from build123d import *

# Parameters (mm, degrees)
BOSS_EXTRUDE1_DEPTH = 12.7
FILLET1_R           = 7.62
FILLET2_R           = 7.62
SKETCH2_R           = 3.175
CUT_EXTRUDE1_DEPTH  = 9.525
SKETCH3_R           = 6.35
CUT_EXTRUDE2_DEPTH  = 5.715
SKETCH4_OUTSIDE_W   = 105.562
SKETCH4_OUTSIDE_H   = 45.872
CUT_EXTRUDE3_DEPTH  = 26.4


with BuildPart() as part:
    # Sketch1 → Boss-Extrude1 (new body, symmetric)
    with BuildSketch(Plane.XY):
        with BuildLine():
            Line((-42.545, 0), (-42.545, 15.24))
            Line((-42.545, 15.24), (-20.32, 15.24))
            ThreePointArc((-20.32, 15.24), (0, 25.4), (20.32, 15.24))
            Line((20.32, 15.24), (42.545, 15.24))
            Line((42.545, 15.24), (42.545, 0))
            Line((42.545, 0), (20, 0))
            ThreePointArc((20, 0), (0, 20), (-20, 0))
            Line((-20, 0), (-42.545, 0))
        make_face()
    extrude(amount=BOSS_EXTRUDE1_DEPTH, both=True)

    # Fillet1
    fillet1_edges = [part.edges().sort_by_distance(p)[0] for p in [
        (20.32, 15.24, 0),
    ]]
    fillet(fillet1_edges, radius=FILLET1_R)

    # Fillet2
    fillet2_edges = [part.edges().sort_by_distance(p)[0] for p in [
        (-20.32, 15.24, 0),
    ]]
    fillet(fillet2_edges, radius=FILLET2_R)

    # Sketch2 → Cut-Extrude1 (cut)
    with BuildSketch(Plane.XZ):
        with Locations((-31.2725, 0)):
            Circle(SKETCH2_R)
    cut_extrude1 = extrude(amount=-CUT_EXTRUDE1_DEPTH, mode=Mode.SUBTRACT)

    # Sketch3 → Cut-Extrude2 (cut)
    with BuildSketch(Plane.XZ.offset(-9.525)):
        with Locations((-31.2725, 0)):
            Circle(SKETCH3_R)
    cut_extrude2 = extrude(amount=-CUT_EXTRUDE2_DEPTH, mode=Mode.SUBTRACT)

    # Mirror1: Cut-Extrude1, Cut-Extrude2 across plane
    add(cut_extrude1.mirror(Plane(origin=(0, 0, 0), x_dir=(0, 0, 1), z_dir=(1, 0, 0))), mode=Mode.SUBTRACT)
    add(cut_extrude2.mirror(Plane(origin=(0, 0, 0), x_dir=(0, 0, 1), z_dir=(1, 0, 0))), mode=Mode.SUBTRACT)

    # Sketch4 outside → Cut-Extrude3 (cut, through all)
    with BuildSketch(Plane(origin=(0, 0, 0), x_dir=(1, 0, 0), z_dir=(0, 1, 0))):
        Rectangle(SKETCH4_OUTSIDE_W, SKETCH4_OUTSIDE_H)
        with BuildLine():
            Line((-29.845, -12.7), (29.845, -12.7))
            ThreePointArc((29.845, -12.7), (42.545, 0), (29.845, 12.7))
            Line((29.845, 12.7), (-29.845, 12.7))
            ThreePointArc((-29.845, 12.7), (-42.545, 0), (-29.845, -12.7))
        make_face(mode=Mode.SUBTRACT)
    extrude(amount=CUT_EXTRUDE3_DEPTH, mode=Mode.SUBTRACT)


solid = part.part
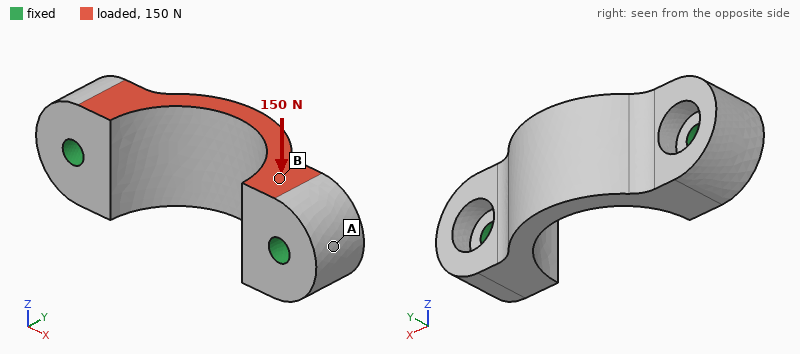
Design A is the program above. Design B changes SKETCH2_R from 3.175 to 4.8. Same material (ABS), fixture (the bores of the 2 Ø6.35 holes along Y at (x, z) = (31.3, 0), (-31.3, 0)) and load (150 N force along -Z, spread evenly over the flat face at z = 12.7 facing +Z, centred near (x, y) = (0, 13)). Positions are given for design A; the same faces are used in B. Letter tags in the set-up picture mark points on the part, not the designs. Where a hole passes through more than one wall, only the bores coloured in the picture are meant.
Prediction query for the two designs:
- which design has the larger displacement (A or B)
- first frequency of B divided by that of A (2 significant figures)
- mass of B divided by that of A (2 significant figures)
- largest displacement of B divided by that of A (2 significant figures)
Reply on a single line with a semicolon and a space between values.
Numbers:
A; 1.3; 0.96; 0.63
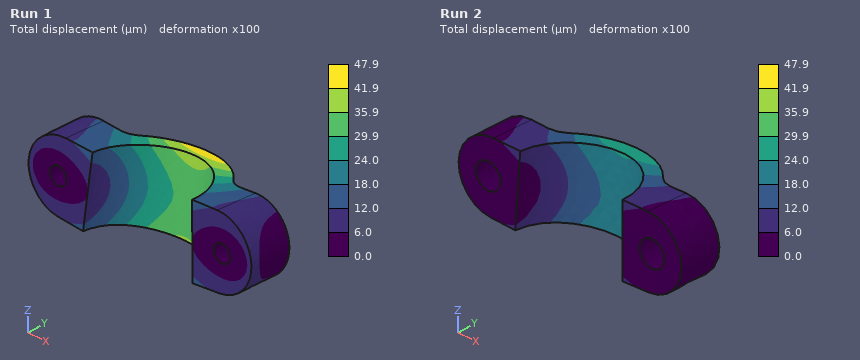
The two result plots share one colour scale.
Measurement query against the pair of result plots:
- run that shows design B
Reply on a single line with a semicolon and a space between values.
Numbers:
Run 2
